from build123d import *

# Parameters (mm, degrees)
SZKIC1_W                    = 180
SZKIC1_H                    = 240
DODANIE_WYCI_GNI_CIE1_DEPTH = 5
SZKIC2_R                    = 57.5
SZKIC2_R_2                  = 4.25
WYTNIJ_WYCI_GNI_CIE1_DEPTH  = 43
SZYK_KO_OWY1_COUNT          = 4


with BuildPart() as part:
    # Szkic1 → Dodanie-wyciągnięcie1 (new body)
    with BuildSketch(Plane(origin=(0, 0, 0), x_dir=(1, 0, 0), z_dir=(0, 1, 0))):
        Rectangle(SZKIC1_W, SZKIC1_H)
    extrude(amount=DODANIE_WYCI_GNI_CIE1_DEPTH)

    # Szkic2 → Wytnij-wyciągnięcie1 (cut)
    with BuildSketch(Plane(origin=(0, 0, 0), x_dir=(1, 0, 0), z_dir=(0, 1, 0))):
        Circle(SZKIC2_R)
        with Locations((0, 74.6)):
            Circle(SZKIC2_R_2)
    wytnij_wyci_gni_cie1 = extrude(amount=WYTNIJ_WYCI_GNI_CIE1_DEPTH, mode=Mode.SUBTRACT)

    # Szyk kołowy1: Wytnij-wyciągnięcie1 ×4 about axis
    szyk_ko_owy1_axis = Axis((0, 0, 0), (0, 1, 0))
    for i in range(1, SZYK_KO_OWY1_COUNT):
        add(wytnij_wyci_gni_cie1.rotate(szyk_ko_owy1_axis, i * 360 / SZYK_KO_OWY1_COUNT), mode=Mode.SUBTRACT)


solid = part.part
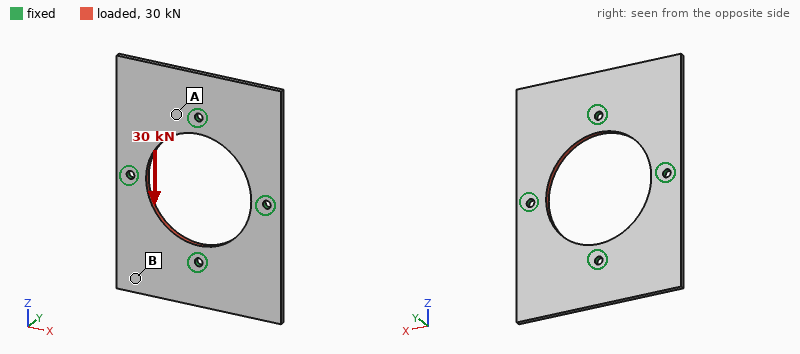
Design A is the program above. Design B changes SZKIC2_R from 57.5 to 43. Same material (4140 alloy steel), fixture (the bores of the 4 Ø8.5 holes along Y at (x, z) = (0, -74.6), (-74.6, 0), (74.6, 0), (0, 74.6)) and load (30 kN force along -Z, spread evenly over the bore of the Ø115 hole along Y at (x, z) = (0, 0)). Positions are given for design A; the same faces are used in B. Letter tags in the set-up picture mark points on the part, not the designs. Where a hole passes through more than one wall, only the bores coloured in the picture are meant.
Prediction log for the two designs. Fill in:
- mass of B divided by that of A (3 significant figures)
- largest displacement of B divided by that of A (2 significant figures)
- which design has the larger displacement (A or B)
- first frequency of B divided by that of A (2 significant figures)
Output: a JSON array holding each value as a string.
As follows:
["1.14", "1.2", "B", "1.1"]
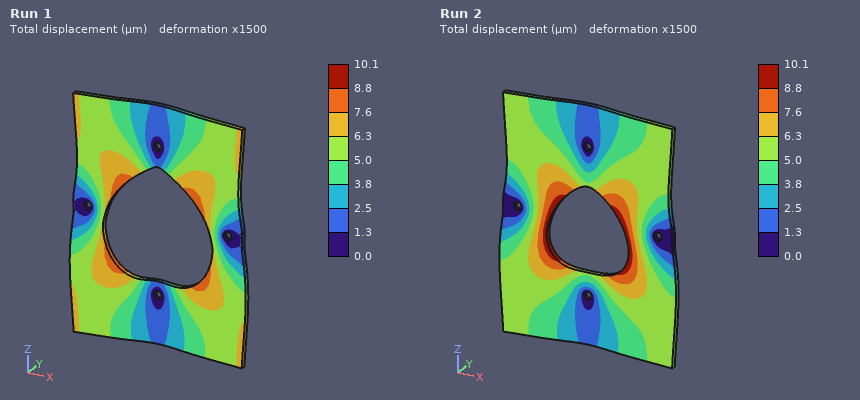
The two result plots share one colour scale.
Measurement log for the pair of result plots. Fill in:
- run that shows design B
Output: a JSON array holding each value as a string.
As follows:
["Run 2"]
